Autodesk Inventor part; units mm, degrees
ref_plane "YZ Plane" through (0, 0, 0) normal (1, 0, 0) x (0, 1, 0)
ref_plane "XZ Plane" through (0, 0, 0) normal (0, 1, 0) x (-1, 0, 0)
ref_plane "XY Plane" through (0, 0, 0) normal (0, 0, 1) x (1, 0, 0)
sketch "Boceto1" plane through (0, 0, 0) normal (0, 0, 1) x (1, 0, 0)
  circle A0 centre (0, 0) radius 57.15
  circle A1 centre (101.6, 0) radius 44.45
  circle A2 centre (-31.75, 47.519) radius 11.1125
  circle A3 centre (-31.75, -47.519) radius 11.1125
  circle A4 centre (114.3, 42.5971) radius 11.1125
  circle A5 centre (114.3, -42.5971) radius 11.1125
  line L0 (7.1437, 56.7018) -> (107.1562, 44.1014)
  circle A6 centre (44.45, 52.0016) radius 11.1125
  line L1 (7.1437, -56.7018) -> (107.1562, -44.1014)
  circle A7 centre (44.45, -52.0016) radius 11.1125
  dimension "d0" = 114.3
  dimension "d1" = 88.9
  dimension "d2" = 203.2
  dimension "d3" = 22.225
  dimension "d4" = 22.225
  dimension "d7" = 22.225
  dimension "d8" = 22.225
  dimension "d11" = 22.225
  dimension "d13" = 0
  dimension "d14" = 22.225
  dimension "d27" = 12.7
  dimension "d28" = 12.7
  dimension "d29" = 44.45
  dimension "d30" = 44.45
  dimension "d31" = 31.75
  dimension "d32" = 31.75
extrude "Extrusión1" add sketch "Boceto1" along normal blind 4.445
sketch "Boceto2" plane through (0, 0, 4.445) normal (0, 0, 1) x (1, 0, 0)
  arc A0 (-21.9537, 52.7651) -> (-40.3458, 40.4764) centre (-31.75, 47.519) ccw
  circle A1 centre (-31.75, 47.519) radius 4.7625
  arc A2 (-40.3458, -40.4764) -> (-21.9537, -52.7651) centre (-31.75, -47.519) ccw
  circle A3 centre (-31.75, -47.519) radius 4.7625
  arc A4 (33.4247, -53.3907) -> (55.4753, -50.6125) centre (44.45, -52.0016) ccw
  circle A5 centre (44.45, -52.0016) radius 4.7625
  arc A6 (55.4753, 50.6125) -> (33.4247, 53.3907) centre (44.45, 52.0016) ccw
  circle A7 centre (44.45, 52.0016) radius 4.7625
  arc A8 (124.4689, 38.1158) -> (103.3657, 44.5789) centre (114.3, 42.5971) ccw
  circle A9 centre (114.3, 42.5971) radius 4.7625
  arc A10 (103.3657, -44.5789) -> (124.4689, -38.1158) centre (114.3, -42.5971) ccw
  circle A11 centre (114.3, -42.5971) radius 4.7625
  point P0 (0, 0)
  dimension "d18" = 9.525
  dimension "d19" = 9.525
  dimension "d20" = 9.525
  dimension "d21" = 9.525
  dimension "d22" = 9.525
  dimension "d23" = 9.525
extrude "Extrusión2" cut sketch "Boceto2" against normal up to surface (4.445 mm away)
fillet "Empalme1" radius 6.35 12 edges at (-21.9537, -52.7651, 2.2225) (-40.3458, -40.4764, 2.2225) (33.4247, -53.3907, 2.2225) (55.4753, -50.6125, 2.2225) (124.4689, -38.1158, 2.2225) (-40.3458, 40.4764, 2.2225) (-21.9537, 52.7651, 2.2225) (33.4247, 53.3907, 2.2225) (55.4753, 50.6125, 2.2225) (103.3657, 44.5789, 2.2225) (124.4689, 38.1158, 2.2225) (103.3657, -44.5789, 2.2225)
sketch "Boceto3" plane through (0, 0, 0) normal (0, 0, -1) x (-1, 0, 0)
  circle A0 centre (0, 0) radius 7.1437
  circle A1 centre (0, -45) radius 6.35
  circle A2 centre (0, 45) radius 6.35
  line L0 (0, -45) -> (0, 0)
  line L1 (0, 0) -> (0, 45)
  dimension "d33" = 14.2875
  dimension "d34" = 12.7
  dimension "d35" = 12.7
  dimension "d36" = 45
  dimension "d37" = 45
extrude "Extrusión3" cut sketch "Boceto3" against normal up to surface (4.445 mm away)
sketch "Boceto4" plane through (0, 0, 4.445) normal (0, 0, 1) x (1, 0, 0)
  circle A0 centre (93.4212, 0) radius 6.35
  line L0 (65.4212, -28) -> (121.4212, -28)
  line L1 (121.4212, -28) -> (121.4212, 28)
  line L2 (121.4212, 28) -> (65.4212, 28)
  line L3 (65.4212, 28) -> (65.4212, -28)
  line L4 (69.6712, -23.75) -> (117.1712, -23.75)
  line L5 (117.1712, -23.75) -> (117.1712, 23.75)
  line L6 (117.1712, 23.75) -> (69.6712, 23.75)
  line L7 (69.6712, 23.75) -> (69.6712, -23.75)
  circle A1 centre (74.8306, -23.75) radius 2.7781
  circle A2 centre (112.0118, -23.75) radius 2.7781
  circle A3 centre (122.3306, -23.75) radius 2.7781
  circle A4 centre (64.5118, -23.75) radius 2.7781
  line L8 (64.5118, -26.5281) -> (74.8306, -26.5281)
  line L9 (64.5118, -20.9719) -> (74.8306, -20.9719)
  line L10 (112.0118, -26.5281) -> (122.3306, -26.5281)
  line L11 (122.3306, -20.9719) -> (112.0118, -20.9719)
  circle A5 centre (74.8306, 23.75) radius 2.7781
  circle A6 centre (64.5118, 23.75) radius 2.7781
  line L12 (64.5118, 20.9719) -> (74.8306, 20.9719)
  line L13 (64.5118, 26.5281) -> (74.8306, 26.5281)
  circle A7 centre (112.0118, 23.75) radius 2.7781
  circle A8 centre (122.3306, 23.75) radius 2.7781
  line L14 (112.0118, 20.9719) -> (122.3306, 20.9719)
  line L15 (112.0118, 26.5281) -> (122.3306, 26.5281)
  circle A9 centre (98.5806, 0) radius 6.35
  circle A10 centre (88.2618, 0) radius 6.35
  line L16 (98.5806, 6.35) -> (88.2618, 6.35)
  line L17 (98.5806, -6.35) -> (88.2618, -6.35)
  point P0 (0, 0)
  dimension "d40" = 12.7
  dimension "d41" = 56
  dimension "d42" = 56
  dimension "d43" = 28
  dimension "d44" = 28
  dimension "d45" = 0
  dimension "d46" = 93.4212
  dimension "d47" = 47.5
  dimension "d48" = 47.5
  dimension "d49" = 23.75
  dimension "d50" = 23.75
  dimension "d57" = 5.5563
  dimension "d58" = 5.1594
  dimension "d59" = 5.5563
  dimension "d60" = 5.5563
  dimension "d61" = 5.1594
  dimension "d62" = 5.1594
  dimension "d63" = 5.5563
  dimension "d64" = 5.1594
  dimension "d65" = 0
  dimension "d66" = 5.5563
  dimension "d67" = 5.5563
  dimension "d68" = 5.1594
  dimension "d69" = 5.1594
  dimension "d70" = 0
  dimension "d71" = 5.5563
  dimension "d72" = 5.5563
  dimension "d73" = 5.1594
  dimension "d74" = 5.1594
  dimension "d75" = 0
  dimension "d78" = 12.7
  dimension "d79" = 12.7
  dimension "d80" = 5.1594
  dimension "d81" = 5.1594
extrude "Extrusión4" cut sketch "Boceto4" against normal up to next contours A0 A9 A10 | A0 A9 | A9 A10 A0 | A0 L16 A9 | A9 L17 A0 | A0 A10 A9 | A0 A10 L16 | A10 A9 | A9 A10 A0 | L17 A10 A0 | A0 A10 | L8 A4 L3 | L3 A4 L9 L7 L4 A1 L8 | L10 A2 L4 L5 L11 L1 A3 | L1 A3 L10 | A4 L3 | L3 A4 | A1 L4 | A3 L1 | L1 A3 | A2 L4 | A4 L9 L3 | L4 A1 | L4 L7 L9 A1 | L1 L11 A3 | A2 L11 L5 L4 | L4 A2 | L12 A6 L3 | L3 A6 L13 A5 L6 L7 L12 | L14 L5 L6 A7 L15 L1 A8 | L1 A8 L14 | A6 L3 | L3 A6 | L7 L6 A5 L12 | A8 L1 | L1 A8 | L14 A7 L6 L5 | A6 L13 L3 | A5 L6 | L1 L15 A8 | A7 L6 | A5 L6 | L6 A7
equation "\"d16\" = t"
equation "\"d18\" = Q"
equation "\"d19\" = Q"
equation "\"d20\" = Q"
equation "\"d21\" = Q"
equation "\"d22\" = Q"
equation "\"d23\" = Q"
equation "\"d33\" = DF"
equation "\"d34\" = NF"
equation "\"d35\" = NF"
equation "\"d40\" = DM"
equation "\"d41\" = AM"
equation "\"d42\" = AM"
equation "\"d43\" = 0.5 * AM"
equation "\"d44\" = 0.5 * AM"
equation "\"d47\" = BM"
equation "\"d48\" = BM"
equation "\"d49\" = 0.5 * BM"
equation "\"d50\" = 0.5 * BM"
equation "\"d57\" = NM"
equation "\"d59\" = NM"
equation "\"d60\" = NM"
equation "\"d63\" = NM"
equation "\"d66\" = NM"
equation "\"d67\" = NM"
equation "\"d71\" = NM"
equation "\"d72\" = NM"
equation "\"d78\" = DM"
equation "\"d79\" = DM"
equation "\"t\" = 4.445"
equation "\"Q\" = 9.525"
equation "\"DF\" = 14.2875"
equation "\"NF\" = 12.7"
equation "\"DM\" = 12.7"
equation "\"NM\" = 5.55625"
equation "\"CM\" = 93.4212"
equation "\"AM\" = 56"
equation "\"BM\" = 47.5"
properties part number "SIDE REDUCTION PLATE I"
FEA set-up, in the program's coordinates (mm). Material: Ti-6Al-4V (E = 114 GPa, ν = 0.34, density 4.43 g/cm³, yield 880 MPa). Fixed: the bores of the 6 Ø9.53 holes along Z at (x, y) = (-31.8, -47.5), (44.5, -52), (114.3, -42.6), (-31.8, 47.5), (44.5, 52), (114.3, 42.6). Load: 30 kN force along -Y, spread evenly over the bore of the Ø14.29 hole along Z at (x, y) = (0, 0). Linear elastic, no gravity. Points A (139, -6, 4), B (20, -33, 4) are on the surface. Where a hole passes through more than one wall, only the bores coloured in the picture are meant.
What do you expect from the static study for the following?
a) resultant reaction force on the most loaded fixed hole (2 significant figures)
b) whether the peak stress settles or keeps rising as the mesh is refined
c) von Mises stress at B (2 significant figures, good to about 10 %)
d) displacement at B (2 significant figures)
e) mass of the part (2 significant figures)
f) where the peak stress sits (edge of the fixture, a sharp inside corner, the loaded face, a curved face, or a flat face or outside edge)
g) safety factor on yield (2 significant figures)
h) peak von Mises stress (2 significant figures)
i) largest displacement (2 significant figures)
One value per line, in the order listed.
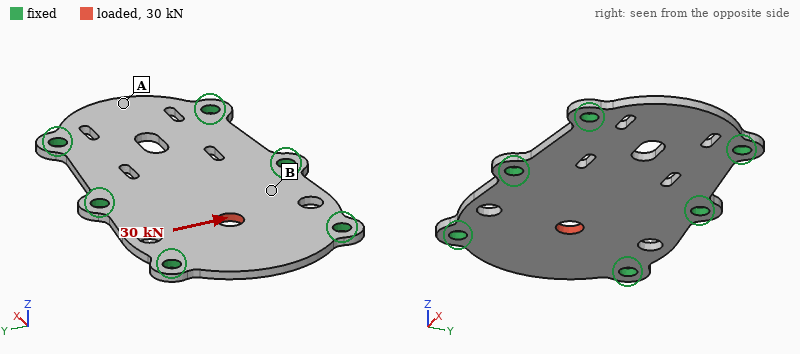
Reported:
9.2 kN
settles
55 MPa
20 µm
360 g
the loaded face
3.3
260 MPa
46 µm
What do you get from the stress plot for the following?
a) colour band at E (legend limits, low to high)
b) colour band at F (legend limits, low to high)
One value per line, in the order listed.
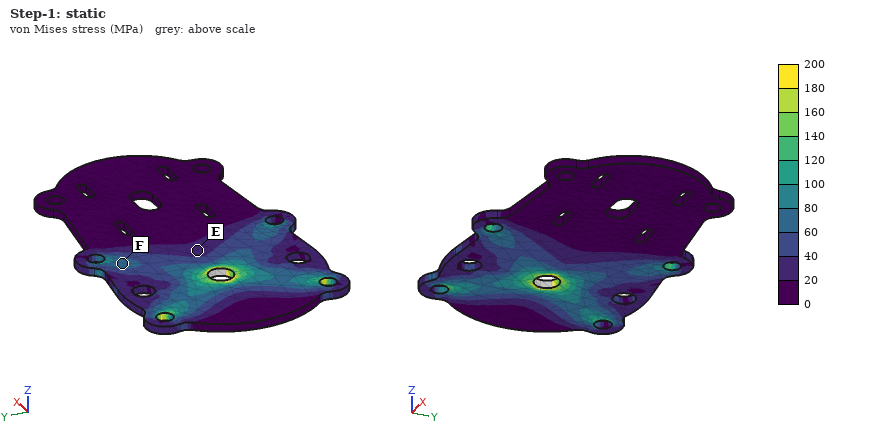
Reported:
20 to 40 MPa
60 to 80 MPa
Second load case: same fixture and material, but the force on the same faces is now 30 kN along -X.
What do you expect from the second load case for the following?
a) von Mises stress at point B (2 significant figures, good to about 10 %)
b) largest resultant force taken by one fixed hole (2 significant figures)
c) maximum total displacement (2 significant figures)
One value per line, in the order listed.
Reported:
50 MPa
7.1 kN
53 µm
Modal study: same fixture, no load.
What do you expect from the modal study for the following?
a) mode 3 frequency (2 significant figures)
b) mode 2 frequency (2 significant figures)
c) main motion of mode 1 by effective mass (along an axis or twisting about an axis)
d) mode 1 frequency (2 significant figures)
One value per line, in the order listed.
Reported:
2500 Hz
2500 Hz
along Z
2100 Hz
